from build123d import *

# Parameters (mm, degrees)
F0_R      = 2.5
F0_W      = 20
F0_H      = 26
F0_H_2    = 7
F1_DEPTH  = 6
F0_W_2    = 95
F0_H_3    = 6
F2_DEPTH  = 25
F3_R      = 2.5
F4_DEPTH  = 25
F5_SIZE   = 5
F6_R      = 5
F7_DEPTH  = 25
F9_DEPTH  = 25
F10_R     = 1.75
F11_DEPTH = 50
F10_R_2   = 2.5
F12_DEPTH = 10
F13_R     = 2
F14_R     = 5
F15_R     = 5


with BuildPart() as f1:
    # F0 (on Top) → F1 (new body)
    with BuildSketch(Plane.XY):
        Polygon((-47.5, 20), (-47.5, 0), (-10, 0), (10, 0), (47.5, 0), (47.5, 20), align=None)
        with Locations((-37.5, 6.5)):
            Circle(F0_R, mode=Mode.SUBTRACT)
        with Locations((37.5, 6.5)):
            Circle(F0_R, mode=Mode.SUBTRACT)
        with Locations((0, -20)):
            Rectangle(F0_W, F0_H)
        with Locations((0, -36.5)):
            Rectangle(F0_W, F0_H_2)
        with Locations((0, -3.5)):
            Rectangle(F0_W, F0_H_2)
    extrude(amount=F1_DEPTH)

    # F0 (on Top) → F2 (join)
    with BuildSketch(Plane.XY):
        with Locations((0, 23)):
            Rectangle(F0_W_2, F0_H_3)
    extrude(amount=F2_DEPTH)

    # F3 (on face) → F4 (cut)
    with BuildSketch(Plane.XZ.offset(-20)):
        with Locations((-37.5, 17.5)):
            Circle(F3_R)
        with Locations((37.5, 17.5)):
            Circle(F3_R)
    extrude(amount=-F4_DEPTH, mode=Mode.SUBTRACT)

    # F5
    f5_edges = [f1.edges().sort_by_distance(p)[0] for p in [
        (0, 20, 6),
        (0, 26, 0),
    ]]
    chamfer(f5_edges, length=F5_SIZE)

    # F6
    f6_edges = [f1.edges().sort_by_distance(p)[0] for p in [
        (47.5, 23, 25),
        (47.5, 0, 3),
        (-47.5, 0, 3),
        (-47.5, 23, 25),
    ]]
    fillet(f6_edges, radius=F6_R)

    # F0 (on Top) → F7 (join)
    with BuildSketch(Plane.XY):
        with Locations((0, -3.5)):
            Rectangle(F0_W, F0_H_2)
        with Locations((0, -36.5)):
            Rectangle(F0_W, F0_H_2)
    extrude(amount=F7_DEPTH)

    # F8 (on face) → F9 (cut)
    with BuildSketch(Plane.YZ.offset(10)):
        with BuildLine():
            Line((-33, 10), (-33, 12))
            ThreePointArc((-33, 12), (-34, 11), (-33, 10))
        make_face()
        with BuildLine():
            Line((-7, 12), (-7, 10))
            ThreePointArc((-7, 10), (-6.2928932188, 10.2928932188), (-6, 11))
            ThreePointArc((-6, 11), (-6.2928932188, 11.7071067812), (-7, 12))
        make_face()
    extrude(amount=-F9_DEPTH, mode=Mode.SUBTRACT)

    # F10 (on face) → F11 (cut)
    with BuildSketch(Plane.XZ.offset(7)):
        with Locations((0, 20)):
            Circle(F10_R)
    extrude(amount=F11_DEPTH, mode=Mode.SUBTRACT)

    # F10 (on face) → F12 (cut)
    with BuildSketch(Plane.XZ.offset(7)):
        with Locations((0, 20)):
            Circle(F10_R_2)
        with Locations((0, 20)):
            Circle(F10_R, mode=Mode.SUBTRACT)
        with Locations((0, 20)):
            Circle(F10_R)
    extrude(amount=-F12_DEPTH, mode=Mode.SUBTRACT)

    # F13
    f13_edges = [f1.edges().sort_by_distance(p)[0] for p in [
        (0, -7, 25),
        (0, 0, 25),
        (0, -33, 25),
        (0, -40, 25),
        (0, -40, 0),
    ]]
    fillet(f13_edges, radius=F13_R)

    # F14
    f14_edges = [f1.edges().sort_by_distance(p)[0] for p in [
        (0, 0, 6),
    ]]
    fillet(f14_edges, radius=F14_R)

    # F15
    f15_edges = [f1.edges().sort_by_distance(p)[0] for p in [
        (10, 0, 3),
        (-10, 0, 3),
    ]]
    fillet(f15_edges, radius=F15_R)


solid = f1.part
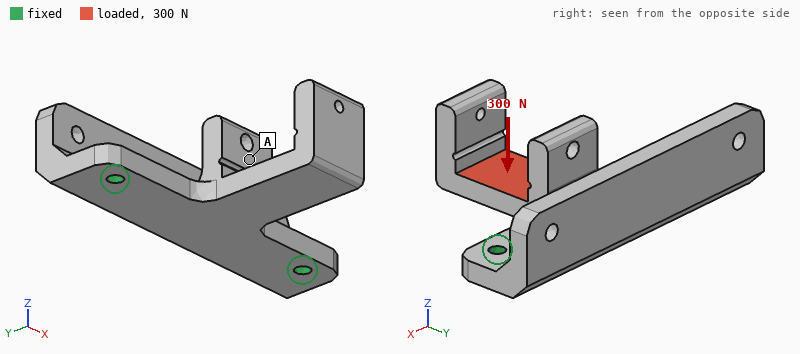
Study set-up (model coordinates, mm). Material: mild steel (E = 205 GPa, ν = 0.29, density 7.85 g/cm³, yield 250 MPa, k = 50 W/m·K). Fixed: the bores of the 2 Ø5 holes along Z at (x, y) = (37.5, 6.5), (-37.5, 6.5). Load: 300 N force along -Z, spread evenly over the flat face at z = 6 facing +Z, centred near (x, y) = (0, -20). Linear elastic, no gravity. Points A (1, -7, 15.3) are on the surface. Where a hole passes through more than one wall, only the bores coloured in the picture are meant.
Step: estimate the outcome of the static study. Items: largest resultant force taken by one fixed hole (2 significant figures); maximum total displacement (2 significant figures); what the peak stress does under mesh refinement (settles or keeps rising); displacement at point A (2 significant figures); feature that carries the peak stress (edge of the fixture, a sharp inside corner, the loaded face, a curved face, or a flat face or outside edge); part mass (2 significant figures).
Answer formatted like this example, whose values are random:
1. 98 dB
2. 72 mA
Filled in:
1. 160 N
2. 98 µm
3. keeps rising
4. 30 µm
5. edge of the fixture
6. 270 g
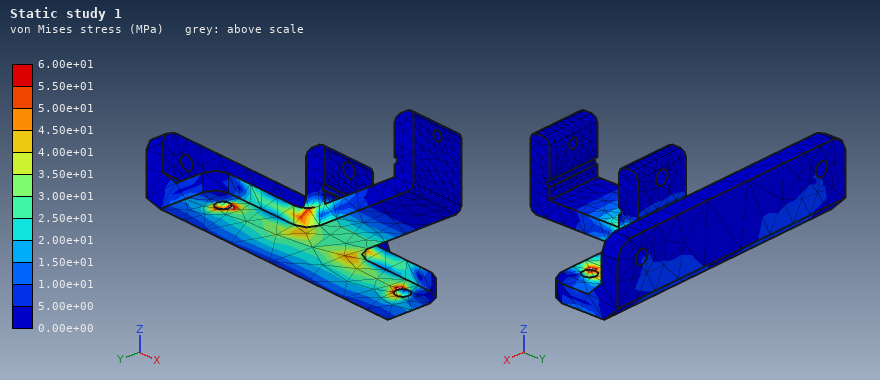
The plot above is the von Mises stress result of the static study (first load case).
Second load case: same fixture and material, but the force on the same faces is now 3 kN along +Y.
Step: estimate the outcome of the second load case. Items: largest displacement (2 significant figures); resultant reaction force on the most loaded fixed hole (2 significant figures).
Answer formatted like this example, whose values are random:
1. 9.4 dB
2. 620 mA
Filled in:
1. 0.14 mm
2. 1.7 kN
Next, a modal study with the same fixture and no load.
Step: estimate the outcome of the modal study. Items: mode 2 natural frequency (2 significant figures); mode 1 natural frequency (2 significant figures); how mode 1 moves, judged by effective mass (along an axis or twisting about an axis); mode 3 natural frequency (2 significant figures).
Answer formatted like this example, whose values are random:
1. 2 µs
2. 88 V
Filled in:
1. 3300 Hz
2. 1100 Hz
3. along Z
4. 3700 Hz
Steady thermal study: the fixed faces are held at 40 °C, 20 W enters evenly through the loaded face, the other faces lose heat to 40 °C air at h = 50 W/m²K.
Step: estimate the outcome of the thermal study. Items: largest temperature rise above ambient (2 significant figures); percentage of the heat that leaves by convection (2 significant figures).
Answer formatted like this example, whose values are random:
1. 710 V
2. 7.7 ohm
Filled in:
1. 61 K
2. 60 %
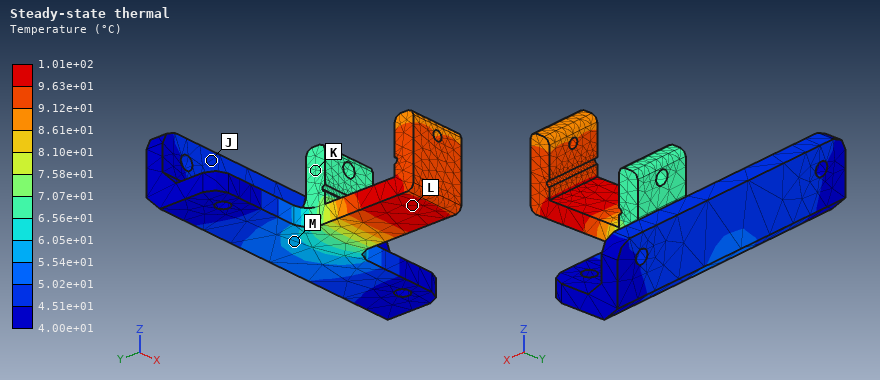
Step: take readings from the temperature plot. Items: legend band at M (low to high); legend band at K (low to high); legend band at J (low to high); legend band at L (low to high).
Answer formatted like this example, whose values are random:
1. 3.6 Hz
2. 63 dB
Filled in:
1. 5.54e+01 to 6.05e+01 °C
2. 6.56e+01 to 7.07e+01 °C
3. 4.51e+01 to 5.02e+01 °C
4. 9.63e+01 to 1.01e+02 °C
